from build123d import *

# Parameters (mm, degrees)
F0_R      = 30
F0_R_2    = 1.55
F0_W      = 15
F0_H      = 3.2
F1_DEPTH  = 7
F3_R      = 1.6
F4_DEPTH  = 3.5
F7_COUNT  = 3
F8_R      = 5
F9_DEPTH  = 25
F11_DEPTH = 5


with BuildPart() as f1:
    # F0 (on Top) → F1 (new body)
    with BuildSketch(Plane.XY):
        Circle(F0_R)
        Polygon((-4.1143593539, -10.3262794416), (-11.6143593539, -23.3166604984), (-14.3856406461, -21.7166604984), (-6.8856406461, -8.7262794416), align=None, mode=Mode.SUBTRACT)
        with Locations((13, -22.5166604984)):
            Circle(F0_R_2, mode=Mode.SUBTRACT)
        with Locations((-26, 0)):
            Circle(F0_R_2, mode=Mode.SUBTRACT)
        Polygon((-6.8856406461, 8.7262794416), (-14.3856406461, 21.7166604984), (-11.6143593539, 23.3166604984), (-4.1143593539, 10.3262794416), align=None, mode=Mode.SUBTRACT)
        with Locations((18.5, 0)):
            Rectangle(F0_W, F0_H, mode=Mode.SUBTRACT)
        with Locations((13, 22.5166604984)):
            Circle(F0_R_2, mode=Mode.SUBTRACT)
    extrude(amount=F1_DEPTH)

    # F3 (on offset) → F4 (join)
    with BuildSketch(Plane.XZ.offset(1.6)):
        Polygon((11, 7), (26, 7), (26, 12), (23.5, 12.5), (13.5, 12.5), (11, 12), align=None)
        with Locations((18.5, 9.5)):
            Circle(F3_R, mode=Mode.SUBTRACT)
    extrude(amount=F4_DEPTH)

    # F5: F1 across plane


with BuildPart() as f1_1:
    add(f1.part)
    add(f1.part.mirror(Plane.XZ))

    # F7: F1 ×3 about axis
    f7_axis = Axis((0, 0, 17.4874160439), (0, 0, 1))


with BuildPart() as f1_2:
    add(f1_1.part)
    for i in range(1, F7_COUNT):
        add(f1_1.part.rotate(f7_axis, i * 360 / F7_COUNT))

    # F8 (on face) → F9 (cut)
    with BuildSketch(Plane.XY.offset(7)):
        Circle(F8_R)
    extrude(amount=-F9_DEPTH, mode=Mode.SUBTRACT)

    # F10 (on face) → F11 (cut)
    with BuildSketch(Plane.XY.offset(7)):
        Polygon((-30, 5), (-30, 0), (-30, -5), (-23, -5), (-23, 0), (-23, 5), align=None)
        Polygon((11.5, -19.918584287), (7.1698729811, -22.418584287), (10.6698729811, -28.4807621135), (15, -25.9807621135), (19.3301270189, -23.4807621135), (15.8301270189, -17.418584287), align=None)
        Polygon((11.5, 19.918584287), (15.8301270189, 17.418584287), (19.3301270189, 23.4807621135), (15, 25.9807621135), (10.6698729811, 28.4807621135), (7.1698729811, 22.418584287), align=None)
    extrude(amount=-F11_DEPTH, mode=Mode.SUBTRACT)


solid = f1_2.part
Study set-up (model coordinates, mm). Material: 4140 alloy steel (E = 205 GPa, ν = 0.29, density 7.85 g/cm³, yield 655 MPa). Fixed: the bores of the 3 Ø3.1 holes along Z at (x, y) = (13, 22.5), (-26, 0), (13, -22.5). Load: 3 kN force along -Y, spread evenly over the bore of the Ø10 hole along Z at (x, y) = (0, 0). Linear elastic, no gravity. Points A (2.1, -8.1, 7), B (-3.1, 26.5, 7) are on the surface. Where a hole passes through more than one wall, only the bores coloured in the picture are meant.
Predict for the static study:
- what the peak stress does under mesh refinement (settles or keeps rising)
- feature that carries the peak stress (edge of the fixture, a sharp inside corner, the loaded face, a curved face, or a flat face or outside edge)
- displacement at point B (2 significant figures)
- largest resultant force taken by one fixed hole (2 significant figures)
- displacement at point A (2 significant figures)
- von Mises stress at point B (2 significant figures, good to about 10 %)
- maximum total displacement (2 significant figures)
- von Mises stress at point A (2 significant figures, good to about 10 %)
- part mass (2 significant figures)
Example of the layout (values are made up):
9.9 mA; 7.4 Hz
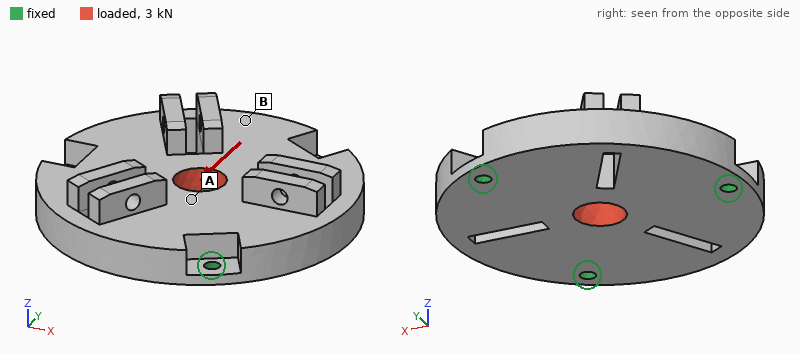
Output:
keeps rising; edge of the fixture; 3.2 µm; 1.1 kN; 2.7 µm; 6.7 MPa; 4.2 µm; 15 MPa; 150 g
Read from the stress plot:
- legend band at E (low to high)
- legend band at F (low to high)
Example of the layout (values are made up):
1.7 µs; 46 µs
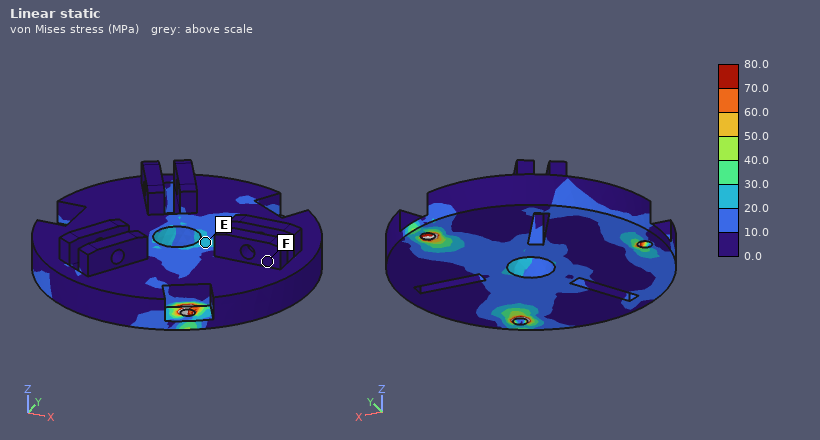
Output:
20.0 to 30.0 MPa; 0.0 to 10.0 MPa
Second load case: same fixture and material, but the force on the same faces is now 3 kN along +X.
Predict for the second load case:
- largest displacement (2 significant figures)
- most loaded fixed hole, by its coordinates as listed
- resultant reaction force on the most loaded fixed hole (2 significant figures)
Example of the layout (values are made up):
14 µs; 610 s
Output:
4.7 µm; (-26, 0); 1.2 kN
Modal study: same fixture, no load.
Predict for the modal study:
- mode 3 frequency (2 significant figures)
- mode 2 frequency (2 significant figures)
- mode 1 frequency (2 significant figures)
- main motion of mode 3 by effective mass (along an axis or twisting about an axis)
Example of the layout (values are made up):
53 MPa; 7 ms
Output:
7400 Hz; 6400 Hz; 6400 Hz; along Z
